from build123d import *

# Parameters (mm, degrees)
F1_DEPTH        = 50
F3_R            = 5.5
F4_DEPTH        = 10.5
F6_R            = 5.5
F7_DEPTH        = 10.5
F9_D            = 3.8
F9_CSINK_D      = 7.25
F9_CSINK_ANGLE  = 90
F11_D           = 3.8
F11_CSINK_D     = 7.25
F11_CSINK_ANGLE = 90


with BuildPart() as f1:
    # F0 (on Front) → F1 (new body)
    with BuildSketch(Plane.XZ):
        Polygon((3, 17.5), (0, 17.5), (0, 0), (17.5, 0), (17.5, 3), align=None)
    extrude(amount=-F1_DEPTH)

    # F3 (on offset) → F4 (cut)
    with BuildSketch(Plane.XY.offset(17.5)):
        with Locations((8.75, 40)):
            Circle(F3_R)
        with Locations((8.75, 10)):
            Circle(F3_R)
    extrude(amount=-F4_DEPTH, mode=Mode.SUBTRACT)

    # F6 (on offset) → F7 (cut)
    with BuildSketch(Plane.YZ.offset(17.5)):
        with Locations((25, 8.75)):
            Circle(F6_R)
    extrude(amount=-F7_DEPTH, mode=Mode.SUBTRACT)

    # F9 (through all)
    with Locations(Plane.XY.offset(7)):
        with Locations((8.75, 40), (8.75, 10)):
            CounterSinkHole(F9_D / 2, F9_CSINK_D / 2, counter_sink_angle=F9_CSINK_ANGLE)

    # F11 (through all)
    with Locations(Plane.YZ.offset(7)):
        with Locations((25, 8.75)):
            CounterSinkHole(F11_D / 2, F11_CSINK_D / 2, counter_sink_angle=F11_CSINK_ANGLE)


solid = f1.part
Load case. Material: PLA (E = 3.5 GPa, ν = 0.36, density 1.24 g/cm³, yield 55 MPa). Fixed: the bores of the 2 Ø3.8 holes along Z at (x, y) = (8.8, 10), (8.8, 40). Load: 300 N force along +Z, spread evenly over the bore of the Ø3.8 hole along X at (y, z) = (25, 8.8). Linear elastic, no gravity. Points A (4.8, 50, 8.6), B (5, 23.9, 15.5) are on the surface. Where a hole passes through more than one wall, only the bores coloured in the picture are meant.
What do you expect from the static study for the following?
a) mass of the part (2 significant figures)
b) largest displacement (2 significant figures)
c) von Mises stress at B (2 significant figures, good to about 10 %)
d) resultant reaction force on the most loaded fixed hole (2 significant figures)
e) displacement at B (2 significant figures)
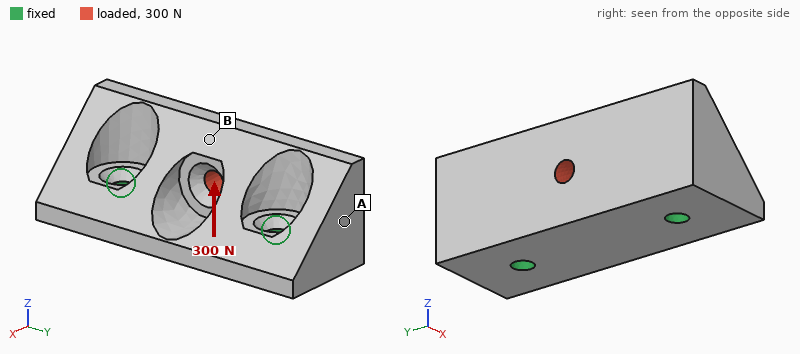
10 g
80 µm
5.7 MPa
160 N
60 µm
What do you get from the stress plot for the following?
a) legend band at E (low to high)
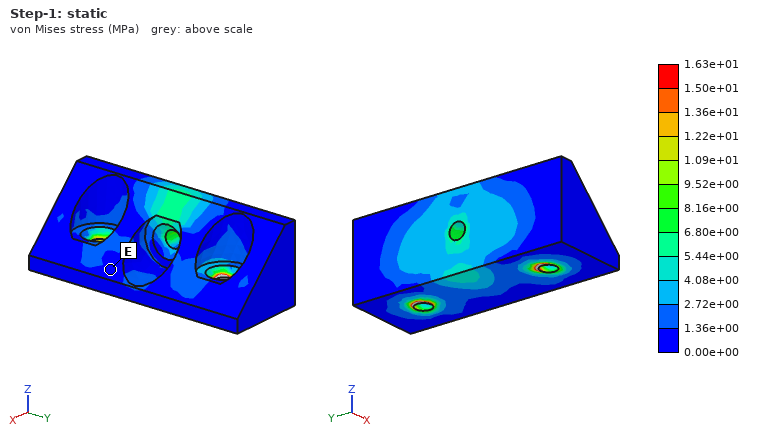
0.00e+00 to 1.36e+00 MPa
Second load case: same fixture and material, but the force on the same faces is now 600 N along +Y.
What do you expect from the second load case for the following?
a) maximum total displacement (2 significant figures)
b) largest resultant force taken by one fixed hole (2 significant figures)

35 µm
340 N
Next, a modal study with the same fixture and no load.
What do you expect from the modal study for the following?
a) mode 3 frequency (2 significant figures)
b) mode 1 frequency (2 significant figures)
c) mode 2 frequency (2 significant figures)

8000 Hz
4900 Hz
6700 Hz
